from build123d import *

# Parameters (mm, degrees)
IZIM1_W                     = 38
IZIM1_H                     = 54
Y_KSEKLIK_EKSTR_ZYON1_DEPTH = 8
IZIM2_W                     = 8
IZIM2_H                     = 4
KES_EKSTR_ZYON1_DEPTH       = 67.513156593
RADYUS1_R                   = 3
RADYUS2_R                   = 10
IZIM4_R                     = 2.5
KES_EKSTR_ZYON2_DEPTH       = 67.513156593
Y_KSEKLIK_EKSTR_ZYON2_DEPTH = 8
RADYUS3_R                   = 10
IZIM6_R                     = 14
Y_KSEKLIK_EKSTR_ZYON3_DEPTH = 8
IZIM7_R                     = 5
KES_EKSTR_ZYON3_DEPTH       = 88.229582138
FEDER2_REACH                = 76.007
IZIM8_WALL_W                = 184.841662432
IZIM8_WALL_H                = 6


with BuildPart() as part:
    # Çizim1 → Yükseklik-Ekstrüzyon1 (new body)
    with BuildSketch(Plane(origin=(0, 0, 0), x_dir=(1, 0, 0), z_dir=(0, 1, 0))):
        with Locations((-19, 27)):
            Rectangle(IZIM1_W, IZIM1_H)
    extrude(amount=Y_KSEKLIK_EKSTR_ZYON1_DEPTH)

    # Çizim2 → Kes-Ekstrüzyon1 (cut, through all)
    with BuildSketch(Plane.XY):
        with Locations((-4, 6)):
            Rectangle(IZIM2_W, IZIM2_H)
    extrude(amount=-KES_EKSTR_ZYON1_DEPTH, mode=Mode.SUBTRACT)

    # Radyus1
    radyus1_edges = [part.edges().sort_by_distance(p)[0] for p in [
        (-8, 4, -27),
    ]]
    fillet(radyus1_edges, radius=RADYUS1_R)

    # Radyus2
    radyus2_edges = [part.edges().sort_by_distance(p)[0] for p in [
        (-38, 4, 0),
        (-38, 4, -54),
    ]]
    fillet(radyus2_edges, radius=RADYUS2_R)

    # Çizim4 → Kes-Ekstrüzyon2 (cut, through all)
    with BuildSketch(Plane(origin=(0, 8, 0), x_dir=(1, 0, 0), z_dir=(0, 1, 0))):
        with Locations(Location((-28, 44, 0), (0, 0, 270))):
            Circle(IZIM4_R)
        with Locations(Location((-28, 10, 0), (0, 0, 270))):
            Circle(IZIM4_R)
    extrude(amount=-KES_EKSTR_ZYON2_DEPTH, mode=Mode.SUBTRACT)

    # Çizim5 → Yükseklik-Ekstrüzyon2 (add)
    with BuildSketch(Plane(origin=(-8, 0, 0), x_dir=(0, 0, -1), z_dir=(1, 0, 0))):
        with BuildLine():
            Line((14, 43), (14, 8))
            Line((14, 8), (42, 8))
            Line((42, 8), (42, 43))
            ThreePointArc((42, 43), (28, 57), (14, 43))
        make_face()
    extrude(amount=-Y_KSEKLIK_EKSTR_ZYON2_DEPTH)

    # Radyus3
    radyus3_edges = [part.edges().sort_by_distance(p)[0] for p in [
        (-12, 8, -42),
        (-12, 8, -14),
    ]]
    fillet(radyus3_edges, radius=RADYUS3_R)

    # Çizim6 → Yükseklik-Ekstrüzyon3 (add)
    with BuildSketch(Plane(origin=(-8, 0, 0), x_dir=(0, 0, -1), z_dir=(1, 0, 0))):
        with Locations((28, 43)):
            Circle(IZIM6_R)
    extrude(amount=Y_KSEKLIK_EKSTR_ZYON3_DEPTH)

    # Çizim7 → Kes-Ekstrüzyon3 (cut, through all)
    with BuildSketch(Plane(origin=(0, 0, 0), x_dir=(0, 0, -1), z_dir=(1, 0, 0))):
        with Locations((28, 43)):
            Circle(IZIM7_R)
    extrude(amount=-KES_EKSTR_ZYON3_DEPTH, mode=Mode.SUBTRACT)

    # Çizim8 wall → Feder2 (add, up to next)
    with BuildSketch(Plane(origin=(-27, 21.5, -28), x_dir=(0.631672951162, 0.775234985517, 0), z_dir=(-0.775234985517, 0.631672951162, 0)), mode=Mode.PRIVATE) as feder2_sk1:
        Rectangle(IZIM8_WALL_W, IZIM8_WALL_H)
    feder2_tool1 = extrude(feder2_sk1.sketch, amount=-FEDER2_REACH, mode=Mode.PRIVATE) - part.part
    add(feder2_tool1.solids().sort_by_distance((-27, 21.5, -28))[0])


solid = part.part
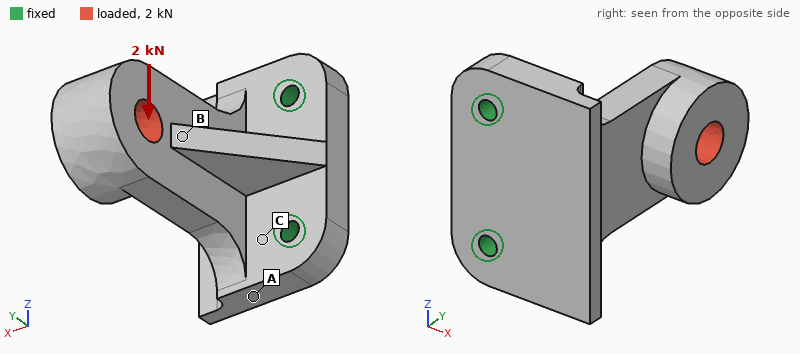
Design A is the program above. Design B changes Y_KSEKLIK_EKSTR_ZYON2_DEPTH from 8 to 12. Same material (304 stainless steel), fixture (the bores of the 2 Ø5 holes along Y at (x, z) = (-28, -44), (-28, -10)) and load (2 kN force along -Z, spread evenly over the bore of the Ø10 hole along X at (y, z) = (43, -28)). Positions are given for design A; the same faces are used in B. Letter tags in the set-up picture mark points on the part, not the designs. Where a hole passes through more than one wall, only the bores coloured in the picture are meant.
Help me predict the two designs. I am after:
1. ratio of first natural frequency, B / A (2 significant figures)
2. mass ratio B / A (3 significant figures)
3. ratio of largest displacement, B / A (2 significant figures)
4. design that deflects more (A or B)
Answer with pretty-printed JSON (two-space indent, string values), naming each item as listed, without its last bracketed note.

{
  "ratio of first natural frequency, B / A": "0.95",
  "mass ratio B / A": "1.15",
  "ratio of largest displacement, B / A": "0.63",
  "design that deflects more": "A"
}
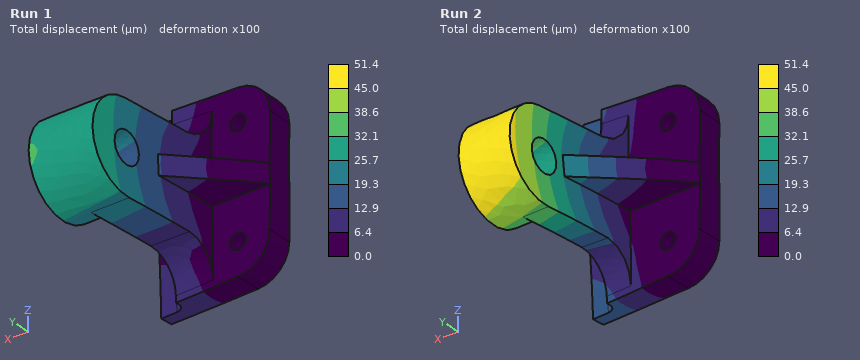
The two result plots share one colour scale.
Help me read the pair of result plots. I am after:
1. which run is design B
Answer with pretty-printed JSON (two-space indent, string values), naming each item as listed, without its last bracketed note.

{
  "which run is design B": "Run 1"
}
